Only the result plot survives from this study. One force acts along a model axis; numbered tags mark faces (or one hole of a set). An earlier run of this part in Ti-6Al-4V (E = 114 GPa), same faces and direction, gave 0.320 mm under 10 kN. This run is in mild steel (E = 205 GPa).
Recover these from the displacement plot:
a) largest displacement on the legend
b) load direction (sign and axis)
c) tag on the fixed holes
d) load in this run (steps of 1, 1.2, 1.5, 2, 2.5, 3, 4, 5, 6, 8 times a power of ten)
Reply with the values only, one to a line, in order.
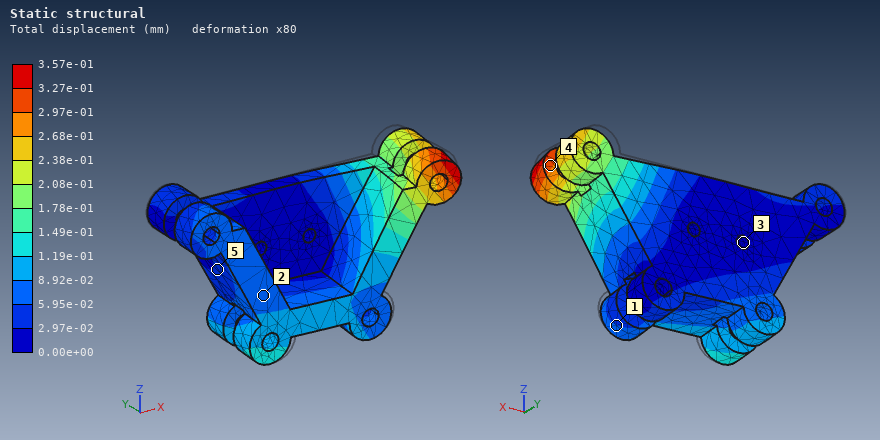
3.57e-01 mm
-Y
3
20 kN
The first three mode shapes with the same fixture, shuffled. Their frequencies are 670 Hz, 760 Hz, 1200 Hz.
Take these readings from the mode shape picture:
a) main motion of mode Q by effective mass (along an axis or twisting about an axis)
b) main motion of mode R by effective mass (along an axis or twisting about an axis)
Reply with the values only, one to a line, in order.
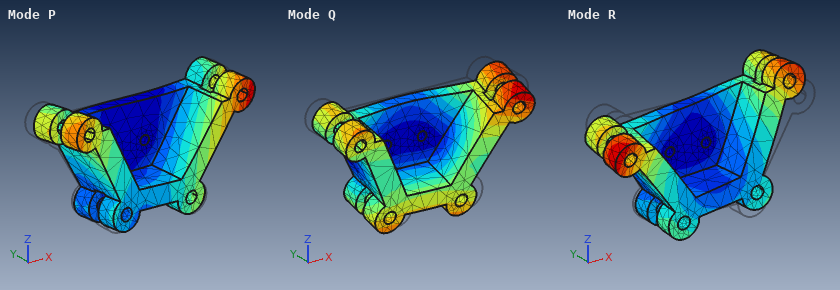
along Z
twisting about Y
